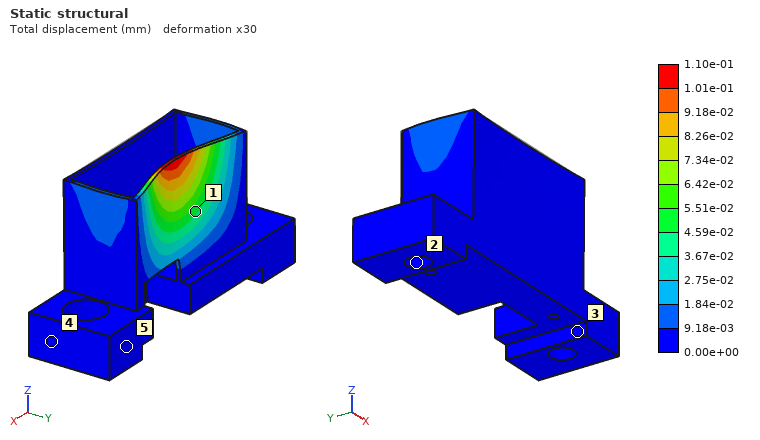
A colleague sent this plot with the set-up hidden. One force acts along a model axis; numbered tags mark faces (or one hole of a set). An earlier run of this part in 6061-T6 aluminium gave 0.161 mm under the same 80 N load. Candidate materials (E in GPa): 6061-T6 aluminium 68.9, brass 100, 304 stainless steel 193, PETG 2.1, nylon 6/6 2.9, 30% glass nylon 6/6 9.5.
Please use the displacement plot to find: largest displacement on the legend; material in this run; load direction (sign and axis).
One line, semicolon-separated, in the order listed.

1.10e-01 mm; brass; -Y
